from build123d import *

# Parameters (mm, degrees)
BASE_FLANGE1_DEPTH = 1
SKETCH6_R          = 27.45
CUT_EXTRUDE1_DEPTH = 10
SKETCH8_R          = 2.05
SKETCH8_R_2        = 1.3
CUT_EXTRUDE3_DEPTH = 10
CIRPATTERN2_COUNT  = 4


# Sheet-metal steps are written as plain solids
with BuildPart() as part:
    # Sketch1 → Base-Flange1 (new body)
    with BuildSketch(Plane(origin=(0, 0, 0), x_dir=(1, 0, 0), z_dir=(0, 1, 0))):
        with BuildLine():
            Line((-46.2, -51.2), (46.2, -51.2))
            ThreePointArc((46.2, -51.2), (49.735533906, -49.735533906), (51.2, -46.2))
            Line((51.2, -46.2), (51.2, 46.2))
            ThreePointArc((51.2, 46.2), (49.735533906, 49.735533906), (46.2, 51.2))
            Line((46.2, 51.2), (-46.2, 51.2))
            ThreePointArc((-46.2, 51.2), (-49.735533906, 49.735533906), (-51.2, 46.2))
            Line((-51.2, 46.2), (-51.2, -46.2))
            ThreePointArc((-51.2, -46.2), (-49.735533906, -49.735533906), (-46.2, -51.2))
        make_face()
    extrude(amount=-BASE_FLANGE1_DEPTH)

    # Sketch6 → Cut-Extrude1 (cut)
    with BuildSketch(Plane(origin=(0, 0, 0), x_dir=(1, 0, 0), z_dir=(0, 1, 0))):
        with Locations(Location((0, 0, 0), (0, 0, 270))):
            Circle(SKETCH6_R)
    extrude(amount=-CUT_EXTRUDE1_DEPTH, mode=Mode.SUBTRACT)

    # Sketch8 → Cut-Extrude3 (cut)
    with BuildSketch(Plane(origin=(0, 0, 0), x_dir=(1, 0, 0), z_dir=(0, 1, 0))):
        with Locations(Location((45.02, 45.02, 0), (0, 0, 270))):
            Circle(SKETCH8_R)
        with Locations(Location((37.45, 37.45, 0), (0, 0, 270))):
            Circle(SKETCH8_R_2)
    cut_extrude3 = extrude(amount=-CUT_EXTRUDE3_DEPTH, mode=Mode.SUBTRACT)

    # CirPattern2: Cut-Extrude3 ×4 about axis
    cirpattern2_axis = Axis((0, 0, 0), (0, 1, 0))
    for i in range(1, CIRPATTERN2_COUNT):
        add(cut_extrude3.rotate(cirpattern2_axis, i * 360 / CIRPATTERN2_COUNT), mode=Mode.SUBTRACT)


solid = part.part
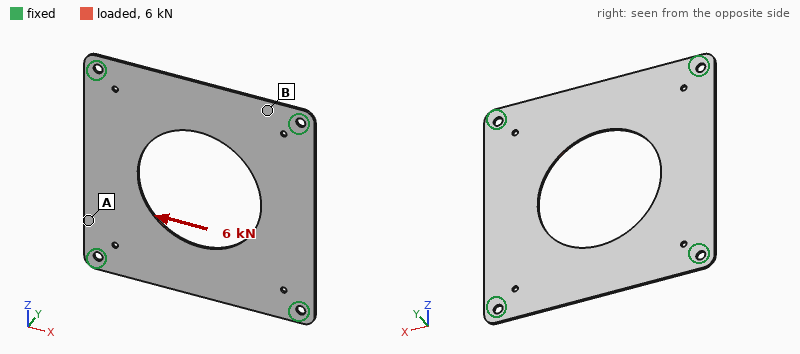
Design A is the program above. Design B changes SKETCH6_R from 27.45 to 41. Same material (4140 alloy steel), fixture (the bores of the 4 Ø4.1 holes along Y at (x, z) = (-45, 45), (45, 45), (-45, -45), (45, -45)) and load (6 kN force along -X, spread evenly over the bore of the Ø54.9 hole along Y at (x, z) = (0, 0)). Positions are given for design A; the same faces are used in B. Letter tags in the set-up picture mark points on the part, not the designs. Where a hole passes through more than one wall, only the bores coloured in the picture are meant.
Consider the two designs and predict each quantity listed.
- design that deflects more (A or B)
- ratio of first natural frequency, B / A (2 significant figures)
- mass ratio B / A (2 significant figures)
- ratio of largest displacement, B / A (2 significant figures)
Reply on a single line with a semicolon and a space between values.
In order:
B; 1.5; 0.64; 3.0
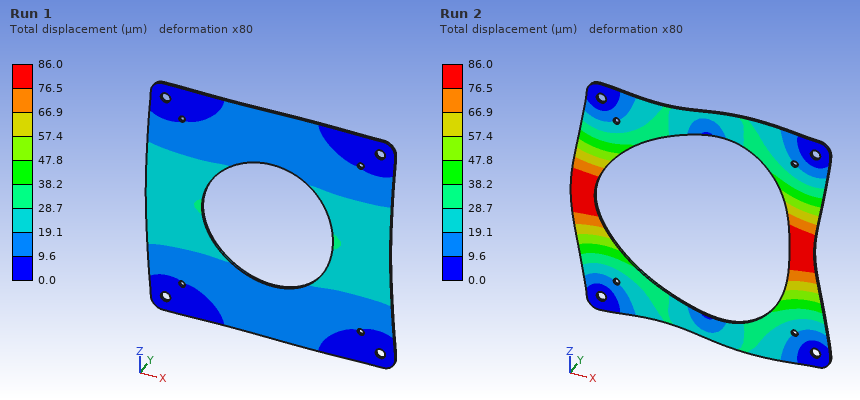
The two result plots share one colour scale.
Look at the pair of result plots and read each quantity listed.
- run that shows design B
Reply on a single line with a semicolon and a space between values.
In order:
Run 2
